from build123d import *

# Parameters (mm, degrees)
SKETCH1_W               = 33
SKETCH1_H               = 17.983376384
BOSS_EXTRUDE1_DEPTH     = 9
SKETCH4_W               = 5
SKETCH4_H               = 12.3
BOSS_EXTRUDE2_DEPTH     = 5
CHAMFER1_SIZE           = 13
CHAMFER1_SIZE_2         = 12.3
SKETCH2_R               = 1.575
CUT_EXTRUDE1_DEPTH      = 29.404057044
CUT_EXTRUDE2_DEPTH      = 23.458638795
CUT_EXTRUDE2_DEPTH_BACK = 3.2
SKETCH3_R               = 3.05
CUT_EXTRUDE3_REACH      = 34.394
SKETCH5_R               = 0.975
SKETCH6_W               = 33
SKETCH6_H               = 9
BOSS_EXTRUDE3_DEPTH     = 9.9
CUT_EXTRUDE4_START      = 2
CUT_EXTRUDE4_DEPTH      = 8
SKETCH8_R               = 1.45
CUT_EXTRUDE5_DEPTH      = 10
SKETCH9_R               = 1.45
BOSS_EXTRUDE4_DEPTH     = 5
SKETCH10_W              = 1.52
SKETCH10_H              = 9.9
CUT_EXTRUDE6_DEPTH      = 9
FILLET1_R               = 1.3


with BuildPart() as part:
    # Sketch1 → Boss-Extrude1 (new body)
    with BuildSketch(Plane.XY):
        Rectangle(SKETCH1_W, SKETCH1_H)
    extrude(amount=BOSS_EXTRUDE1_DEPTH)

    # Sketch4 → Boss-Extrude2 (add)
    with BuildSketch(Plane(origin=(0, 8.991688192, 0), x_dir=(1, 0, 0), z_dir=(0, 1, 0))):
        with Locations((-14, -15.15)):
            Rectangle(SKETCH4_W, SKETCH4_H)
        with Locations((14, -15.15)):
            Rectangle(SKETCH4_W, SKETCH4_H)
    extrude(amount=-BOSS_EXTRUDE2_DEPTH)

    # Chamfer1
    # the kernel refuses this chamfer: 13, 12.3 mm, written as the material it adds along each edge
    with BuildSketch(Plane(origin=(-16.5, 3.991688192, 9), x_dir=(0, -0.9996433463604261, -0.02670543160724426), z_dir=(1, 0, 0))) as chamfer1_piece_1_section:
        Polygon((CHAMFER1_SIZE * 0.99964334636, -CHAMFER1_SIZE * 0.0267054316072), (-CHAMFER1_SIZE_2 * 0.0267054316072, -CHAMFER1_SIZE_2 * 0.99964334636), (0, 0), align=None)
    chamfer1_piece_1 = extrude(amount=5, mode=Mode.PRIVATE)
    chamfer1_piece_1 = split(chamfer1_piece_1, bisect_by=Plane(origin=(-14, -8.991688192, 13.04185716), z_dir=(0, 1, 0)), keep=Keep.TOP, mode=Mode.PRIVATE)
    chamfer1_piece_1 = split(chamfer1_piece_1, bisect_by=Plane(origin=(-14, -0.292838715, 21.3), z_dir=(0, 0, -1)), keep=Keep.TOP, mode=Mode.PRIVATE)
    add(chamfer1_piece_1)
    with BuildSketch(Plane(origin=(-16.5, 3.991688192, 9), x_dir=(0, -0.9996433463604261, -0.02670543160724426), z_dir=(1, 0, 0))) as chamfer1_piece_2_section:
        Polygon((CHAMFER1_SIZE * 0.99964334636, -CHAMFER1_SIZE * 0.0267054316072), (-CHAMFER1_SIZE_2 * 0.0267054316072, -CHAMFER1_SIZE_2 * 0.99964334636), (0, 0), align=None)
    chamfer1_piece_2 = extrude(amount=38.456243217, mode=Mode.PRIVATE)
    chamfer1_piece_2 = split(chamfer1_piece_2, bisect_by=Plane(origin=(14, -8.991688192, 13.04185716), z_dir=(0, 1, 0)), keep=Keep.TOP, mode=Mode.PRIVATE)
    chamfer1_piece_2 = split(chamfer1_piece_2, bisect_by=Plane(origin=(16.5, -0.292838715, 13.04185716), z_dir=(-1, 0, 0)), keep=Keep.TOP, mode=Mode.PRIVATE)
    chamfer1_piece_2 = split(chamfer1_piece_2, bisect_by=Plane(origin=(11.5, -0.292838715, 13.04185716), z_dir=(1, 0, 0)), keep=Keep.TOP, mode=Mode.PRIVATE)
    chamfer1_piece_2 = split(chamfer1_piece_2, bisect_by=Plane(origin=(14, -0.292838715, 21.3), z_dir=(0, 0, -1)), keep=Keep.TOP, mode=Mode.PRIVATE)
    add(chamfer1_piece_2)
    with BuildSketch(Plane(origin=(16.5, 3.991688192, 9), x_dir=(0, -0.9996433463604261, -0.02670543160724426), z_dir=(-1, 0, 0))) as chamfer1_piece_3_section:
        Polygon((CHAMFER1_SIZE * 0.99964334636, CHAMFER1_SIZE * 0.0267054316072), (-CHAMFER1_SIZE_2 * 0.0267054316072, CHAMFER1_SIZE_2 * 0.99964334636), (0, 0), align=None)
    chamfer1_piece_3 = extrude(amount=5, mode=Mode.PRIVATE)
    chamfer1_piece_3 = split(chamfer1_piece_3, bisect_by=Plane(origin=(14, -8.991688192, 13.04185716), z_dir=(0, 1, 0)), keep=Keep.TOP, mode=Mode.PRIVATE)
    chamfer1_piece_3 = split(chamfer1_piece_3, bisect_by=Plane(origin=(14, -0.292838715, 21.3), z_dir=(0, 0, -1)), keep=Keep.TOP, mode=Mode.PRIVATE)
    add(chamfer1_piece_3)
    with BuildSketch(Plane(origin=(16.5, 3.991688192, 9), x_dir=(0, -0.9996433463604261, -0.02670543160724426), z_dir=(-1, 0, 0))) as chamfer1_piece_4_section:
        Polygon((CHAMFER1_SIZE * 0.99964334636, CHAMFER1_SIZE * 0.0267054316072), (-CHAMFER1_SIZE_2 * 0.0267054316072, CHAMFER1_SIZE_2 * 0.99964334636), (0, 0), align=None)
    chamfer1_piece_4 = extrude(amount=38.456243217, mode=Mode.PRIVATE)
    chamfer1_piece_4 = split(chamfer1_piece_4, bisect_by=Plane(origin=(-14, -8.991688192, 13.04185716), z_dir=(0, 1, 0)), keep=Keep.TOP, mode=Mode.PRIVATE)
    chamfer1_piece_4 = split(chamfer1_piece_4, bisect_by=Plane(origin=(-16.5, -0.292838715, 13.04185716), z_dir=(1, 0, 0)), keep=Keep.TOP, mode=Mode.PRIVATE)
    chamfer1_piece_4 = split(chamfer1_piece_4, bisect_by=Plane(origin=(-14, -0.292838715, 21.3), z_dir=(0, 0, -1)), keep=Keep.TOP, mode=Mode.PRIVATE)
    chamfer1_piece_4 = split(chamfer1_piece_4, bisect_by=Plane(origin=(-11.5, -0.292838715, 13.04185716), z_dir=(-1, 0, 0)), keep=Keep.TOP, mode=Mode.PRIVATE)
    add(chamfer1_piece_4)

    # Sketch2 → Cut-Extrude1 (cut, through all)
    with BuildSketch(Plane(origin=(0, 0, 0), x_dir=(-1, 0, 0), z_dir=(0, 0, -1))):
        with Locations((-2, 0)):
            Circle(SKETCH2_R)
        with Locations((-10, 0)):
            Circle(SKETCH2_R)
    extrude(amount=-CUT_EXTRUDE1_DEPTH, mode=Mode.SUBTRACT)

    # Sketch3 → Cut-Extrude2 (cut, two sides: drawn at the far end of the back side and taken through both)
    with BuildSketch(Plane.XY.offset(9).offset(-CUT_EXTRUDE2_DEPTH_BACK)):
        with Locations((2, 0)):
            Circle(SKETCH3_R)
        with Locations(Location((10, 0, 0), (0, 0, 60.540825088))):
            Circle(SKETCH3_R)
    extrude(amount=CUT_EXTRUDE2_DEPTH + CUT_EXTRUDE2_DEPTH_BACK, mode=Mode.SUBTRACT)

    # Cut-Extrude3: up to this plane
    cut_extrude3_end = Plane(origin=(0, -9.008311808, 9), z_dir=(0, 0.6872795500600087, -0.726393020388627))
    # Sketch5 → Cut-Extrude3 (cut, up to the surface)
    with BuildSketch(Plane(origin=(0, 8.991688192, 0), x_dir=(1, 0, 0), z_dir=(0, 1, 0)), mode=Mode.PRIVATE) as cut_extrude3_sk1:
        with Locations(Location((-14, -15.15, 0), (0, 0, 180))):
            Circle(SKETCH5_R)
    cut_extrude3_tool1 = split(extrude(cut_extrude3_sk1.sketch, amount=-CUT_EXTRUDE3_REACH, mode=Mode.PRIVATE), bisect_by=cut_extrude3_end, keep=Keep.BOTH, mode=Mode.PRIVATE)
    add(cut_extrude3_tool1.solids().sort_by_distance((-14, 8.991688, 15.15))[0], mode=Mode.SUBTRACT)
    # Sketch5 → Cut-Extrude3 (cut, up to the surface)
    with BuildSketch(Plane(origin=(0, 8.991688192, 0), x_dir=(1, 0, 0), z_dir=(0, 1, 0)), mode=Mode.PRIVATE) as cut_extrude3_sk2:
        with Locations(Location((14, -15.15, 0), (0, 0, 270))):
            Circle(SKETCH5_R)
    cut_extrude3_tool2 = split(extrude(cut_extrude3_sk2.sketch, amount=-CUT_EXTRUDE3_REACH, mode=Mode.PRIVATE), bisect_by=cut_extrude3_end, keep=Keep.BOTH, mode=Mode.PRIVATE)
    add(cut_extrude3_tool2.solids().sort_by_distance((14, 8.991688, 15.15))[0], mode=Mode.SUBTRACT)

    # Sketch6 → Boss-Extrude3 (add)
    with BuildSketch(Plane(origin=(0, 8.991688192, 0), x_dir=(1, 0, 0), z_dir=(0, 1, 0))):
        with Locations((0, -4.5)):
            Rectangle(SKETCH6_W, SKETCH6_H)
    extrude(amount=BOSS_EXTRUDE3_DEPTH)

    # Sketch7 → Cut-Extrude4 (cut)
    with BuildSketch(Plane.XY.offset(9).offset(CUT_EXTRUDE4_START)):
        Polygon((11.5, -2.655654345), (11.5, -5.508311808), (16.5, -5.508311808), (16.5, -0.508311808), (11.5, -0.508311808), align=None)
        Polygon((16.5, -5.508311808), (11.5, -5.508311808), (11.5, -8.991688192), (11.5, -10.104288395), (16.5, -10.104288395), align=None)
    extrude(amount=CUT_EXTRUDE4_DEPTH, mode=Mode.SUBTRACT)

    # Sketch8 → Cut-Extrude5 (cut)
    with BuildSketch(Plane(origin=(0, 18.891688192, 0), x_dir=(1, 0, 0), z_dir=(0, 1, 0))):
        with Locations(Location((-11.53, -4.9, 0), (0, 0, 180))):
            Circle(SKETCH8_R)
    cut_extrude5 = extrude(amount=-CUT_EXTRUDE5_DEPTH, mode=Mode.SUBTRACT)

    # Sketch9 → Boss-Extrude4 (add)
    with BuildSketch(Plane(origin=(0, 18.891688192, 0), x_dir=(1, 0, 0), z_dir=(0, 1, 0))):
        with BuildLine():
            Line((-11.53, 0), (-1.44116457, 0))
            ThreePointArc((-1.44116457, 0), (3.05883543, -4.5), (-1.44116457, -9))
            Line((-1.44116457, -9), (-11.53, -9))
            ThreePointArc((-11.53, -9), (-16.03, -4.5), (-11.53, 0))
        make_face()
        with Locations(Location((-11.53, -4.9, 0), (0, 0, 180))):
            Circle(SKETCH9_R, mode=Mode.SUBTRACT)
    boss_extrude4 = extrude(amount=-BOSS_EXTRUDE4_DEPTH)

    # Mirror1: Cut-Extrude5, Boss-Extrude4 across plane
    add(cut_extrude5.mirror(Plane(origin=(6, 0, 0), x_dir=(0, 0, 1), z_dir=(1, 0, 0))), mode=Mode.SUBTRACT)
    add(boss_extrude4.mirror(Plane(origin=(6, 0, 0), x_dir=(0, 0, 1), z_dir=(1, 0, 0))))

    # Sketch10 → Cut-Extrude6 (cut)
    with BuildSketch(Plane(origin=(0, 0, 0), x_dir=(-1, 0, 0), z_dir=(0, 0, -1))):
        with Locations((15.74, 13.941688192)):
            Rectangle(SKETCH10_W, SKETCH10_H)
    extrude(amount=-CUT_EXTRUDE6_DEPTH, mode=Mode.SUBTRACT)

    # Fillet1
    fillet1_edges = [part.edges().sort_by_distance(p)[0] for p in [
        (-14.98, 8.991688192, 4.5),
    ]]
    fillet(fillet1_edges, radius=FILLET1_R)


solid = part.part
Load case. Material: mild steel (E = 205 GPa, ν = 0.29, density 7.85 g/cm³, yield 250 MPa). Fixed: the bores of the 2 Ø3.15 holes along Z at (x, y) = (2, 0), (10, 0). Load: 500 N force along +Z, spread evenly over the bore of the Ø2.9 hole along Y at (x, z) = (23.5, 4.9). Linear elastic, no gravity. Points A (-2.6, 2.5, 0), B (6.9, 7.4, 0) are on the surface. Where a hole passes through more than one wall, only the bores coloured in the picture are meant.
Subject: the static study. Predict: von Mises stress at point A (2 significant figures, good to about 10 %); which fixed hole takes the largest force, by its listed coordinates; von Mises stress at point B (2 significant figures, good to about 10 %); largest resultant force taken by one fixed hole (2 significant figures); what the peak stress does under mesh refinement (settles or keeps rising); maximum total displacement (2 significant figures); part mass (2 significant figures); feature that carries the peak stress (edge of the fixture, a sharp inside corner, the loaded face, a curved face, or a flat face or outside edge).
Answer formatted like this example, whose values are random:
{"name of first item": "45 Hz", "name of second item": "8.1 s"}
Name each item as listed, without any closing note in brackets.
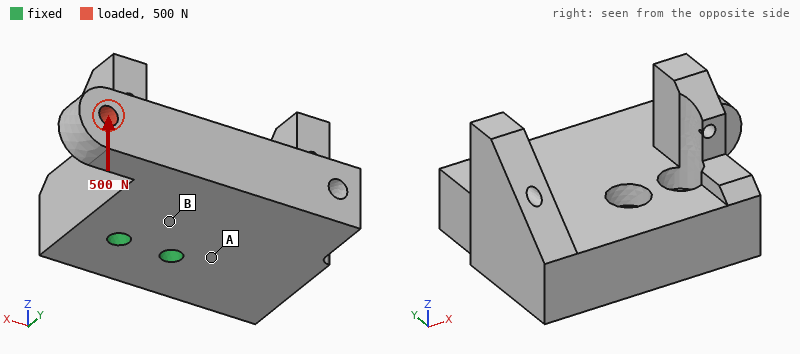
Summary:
{"von Mises stress at point A": "9.5 MPa", "which fixed hole takes the largest force, by its listed coordinates": "(10, 0)", "von Mises stress at point B": "31 MPa", "largest resultant force taken by one fixed hole": "880 N", "what the peak stress does under mesh refinement": "keeps rising", "maximum total displacement": "25 µm", "part mass": "74 g", "feature that carries the peak stress": "edge of the fixture"}
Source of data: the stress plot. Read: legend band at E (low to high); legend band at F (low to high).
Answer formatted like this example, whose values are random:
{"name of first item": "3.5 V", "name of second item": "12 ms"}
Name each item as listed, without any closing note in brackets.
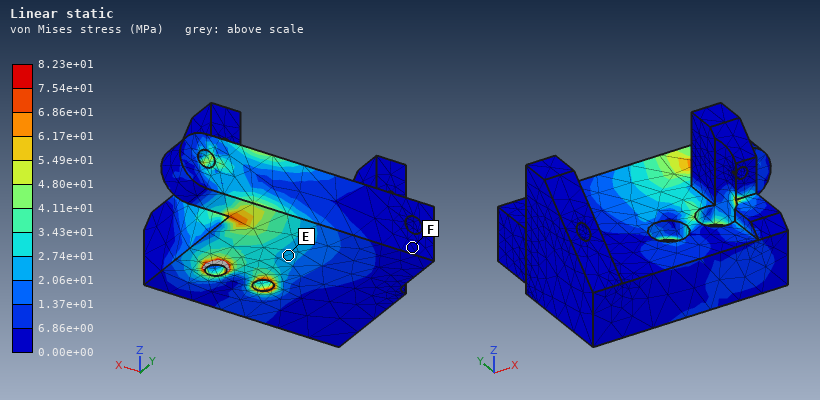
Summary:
{"legend band at E": "2.06e+01 to 2.74e+01 MPa", "legend band at F": "0.00e+00 to 6.86e+00 MPa"}
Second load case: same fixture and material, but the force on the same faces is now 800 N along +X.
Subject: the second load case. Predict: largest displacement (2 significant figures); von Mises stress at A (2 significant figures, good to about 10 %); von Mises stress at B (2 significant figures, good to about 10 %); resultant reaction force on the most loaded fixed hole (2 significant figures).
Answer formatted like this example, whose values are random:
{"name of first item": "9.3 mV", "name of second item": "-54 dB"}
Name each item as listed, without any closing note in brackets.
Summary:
{"largest displacement": "7.1 µm", "von Mises stress at A": "7.2 MPa", "von Mises stress at B": "15 MPa", "resultant reaction force on the most loaded fixed hole": "1.3 kN"}
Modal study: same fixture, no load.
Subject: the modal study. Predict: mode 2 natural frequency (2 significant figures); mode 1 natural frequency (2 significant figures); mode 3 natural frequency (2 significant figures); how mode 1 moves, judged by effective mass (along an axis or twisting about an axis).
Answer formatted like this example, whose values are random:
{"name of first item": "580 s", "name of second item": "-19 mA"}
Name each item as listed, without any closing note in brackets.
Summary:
{"mode 2 natural frequency": "9600 Hz", "mode 1 natural frequency": "8700 Hz", "mode 3 natural frequency": "11 kHz", "how mode 1 moves, judged by effective mass": "along Z"}
